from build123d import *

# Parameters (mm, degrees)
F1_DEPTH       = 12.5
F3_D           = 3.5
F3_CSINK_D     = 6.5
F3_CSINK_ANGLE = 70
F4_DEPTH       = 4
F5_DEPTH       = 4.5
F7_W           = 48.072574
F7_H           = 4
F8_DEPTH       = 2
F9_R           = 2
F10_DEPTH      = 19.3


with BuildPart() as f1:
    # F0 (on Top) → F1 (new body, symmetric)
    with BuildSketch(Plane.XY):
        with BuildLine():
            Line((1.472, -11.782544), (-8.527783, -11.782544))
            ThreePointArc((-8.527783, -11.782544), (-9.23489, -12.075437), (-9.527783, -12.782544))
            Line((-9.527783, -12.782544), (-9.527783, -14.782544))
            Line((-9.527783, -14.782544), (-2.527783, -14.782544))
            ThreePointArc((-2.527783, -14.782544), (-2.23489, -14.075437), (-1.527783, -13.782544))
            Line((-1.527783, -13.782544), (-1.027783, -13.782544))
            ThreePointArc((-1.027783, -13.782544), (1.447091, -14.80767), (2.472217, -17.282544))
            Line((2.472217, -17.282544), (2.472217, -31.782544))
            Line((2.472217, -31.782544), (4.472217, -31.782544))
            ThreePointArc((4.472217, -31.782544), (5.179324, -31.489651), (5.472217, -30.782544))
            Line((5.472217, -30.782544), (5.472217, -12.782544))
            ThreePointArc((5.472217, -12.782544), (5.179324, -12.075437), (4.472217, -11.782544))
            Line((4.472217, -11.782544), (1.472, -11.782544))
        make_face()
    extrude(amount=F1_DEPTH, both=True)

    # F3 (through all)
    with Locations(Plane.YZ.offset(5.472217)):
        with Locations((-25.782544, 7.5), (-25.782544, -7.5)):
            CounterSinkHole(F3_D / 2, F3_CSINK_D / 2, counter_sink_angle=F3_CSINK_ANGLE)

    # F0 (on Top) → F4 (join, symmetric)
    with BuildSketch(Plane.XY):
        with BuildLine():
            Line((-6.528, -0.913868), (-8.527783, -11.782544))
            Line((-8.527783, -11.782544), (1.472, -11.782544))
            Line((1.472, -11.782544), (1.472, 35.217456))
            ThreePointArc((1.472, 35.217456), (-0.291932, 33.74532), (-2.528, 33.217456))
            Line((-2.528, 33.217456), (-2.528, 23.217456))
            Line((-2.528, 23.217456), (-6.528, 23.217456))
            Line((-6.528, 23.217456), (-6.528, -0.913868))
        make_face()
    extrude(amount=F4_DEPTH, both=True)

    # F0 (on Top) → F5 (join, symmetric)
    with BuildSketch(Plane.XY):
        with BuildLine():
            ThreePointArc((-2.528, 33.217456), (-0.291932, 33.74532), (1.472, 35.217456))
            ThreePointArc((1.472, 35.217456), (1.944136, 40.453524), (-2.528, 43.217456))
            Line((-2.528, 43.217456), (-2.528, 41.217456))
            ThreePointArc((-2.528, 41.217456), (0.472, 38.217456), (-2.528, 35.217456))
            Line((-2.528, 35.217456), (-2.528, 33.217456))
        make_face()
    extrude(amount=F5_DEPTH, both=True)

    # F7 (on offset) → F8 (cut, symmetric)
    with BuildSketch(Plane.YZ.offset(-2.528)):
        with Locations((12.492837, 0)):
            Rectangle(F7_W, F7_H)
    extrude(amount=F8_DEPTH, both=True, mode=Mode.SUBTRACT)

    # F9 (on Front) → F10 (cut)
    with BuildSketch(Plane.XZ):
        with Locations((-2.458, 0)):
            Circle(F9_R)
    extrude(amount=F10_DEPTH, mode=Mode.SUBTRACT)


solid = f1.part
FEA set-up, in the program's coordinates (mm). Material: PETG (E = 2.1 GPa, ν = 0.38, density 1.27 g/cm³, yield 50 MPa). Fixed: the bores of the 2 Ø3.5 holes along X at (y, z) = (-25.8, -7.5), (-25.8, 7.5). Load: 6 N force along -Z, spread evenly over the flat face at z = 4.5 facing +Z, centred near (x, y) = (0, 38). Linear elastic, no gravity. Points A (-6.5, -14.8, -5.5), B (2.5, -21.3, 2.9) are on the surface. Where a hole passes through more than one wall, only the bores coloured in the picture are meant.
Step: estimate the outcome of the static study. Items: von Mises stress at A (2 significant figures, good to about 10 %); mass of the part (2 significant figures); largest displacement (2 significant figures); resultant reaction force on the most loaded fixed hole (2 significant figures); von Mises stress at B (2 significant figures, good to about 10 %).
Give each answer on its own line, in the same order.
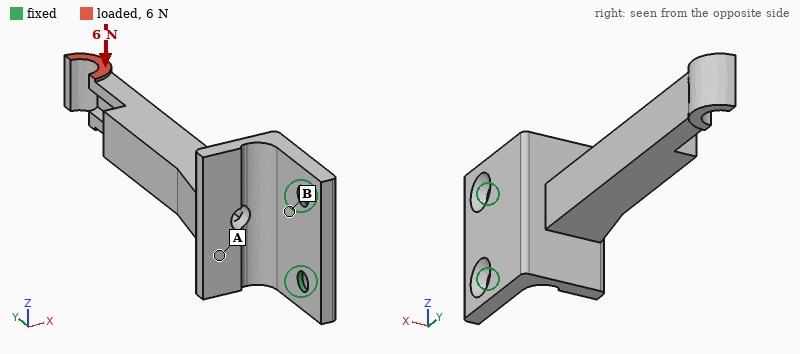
2.7 MPa
5.6 g
0.83 mm
23 N
0.86 MPa
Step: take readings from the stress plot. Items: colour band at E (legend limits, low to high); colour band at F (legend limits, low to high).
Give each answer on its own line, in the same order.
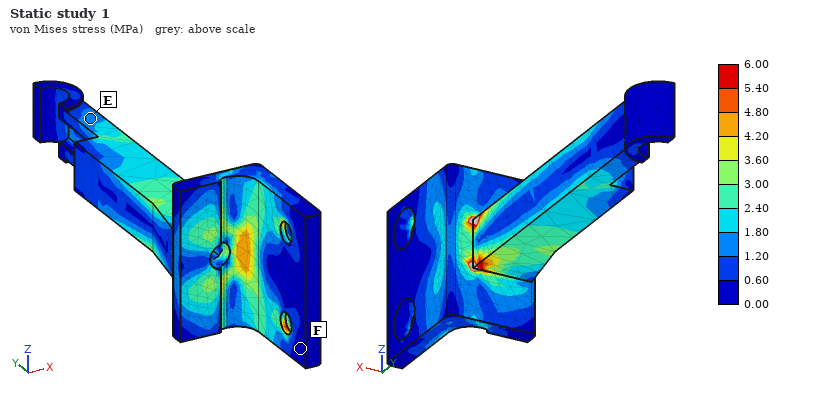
1.20 to 1.80 MPa
0.00 to 0.60 MPa
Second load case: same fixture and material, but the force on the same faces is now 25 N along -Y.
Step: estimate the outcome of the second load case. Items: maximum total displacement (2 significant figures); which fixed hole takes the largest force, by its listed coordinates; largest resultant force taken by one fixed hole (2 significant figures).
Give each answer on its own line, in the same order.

0.83 mm
(-25.8, 7.5)
20 N
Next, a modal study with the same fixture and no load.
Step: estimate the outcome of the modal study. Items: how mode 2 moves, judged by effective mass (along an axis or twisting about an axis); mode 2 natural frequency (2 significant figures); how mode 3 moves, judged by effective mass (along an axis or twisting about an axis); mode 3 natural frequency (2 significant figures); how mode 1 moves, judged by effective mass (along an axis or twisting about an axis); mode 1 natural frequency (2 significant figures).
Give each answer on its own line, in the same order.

along Z
550 Hz
along X
1300 Hz
along X
190 Hz
